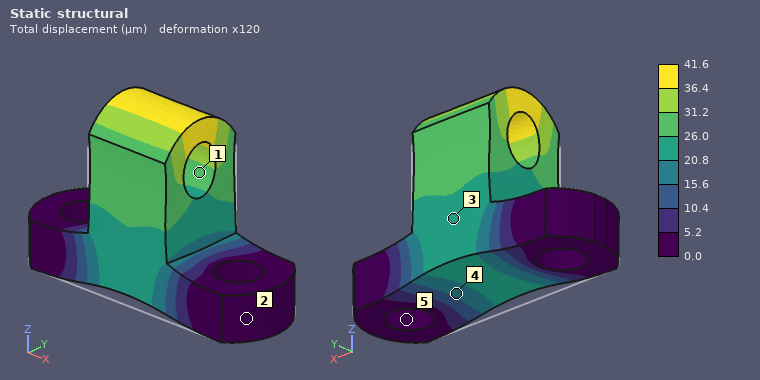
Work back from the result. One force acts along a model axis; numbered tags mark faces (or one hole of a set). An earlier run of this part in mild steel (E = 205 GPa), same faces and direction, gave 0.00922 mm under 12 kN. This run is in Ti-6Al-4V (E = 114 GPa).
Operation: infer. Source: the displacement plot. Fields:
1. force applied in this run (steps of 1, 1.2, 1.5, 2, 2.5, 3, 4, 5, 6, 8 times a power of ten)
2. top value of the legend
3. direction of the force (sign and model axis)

30 kN
41.6 µm
+Z
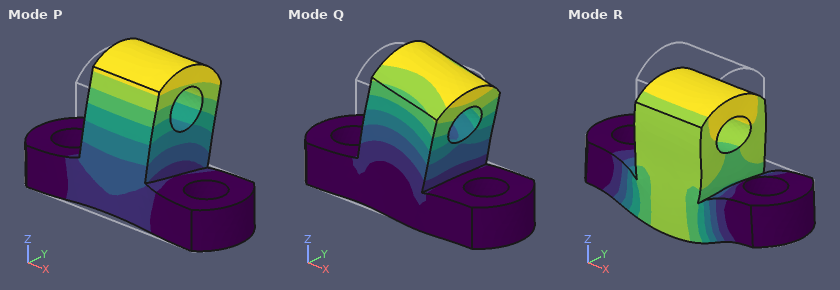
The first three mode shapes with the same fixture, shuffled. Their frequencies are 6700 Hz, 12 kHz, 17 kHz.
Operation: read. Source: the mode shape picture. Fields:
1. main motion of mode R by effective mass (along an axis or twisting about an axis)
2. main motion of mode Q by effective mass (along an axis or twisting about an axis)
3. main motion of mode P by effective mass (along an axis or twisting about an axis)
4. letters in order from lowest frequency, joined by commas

along Z
along X
along Y
P, Q, R
